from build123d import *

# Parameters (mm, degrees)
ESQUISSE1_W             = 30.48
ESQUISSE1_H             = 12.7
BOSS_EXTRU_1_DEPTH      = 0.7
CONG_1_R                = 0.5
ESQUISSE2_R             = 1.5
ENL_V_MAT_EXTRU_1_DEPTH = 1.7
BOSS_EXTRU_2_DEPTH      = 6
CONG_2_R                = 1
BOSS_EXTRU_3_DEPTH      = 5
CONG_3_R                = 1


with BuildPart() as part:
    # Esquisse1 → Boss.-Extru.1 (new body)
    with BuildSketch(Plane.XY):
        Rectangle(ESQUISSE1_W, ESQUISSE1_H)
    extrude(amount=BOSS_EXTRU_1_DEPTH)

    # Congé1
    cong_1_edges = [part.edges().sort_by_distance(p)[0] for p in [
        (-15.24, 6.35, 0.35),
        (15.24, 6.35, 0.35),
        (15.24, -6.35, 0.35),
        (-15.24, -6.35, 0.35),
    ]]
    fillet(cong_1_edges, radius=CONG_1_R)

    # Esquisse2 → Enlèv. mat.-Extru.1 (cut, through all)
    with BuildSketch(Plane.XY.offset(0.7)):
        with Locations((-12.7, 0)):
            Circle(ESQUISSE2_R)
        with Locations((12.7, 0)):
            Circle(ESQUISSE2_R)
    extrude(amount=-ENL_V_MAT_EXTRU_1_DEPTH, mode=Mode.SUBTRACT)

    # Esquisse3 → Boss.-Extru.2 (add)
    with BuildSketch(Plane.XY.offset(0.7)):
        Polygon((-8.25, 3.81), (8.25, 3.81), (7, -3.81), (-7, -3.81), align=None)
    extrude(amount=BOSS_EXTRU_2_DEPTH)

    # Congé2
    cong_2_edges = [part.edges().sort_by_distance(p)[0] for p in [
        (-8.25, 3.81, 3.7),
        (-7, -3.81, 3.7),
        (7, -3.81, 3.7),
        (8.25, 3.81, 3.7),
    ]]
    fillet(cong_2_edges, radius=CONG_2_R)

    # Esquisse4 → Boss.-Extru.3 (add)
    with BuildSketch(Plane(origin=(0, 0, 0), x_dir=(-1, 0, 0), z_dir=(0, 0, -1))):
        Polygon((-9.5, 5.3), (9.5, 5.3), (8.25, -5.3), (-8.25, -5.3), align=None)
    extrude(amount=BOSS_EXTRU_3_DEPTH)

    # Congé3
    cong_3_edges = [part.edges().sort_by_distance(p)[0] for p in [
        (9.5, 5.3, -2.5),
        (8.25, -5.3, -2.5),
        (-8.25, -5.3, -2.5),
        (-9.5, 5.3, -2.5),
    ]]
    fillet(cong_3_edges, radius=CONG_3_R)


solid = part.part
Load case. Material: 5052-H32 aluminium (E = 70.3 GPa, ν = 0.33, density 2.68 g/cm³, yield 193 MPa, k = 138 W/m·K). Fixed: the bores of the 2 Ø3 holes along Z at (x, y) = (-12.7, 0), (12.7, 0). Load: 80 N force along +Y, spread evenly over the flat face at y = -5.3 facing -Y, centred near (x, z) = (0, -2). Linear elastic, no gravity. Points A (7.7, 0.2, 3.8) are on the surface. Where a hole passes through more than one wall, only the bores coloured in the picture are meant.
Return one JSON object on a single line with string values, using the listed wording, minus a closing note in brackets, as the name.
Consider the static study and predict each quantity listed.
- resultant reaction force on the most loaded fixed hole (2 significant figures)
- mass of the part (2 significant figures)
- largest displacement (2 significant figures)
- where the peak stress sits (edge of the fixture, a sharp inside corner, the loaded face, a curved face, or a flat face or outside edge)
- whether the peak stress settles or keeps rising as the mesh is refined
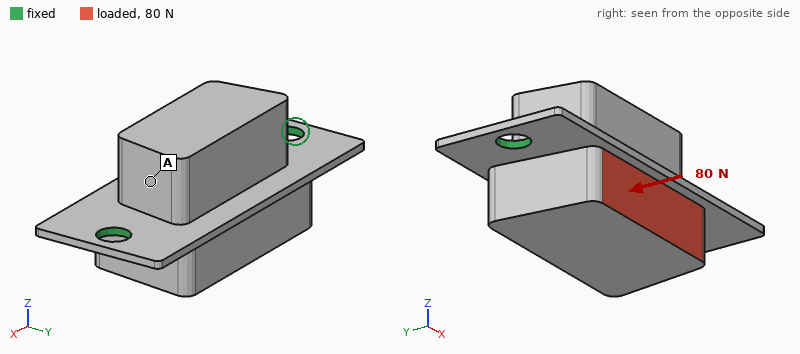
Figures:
{"resultant reaction force on the most loaded fixed hole": "40 N", "mass of the part": "5.1 g", "largest displacement": "38 µm", "where the peak stress sits": "edge of the fixture", "whether the peak stress settles or keeps rising as the mesh is refined": "keeps rising"}
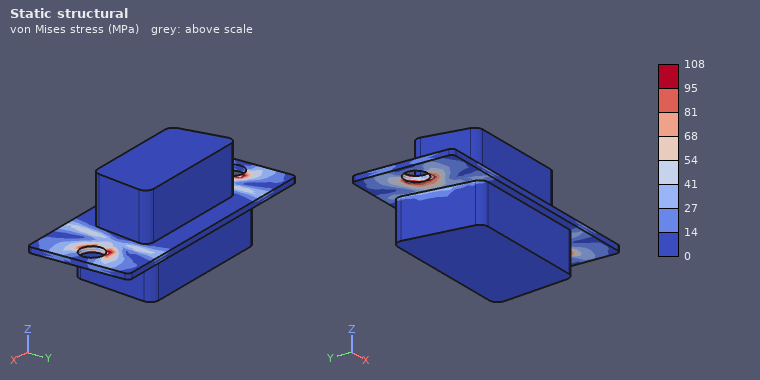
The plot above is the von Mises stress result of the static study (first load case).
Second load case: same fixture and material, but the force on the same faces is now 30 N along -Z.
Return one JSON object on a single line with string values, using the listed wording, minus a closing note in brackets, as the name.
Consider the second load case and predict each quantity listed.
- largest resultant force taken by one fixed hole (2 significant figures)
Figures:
{"largest resultant force taken by one fixed hole": "17 N"}
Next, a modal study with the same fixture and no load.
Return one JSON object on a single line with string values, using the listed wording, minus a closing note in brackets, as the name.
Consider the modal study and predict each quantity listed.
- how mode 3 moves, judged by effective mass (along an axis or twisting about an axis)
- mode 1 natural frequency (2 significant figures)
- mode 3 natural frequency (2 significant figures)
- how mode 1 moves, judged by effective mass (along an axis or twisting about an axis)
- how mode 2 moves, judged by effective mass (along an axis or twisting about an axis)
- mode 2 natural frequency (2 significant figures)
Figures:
{"how mode 3 moves, judged by effective mass": "twisting about Y", "mode 1 natural frequency": "3600 Hz", "mode 3 natural frequency": "13 kHz", "how mode 1 moves, judged by effective mass": "twisting about X", "how mode 2 moves, judged by effective mass": "along Z", "mode 2 natural frequency": "7400 Hz"}
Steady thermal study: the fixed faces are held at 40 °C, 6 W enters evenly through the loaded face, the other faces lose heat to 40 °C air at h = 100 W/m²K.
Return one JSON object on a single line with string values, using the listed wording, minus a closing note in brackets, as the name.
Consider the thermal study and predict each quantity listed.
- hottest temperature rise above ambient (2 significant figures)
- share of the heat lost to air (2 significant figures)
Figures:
{"hottest temperature rise above ambient": "13 K", "share of the heat lost to air": "19 %"}
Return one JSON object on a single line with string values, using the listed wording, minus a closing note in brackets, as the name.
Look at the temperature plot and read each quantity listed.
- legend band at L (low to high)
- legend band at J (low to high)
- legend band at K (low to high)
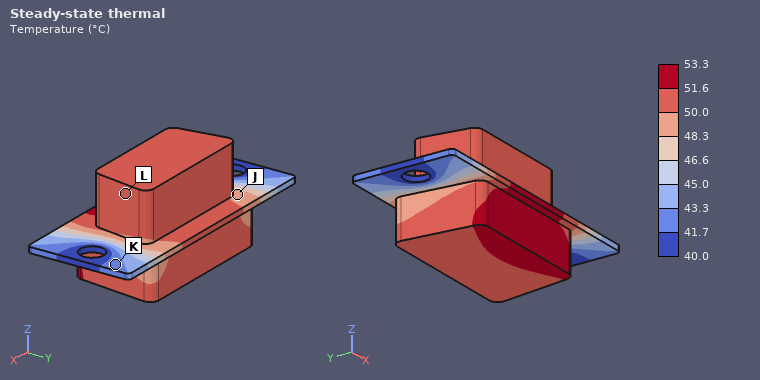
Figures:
{"legend band at L": "50.0 to 51.6 °C", "legend band at J": "48.3 to 50.0 °C", "legend band at K": "41.7 to 43.3 °C"}
